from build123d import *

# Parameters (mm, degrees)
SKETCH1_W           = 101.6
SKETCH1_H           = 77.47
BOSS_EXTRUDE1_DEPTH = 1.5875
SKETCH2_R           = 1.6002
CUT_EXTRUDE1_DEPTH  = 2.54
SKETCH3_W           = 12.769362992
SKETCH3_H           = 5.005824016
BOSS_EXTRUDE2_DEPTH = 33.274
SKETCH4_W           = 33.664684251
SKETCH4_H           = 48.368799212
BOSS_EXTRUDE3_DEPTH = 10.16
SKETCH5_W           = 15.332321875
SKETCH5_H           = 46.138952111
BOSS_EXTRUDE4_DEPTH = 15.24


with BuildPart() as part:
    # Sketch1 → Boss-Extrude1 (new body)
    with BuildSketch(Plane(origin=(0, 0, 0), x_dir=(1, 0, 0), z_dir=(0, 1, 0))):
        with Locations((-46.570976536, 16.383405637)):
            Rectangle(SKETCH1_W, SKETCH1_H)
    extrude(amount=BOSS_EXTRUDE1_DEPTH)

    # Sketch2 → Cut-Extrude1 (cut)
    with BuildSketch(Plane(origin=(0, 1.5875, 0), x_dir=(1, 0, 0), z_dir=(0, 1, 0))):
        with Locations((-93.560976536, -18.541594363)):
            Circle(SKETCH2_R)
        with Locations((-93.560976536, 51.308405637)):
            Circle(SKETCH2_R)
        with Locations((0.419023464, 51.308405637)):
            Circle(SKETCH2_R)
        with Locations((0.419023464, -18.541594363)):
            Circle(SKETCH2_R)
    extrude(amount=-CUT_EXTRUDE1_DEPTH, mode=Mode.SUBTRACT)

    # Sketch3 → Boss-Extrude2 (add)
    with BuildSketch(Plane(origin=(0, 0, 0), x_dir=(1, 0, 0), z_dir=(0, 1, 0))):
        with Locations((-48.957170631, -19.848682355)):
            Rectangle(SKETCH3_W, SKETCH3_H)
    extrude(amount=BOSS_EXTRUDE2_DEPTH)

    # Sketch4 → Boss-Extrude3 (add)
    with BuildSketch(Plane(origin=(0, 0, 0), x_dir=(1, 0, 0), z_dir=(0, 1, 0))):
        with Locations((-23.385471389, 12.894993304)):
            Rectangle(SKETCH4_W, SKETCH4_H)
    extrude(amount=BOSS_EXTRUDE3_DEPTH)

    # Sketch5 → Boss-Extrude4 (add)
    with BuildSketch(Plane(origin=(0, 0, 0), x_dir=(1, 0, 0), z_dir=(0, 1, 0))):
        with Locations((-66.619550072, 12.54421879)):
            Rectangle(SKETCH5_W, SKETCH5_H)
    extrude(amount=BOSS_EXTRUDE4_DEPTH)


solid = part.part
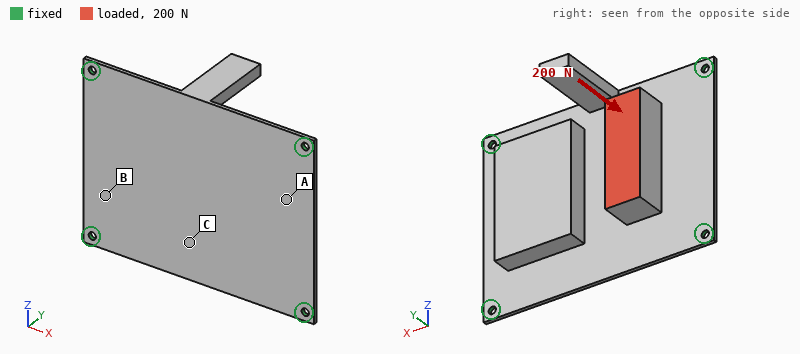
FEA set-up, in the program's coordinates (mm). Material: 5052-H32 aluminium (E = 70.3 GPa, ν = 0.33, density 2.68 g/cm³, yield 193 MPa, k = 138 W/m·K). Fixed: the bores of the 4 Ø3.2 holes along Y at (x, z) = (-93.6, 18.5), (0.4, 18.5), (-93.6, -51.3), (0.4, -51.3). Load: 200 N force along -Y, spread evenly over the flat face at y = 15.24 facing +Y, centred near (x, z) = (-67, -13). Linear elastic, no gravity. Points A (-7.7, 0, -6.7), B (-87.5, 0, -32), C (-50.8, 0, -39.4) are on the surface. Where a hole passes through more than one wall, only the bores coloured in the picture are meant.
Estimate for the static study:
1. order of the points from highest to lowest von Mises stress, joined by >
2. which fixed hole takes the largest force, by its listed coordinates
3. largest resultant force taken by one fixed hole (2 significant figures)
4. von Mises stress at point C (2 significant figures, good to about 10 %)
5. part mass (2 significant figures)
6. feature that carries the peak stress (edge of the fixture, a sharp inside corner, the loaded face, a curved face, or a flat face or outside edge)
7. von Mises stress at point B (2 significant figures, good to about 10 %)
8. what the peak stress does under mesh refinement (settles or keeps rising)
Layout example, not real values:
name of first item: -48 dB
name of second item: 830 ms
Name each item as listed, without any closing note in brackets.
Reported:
order of the points from highest to lowest von Mises stress, joined by >: C > B > A
which fixed hole takes the largest force, by its listed coordinates: (-93.6, 18.5)
largest resultant force taken by one fixed hole: 92 N
von Mises stress at point C: 38 MPa
part mass: 100 g
feature that carries the peak stress: edge of the fixture
von Mises stress at point B: 20 MPa
what the peak stress does under mesh refinement: keeps rising
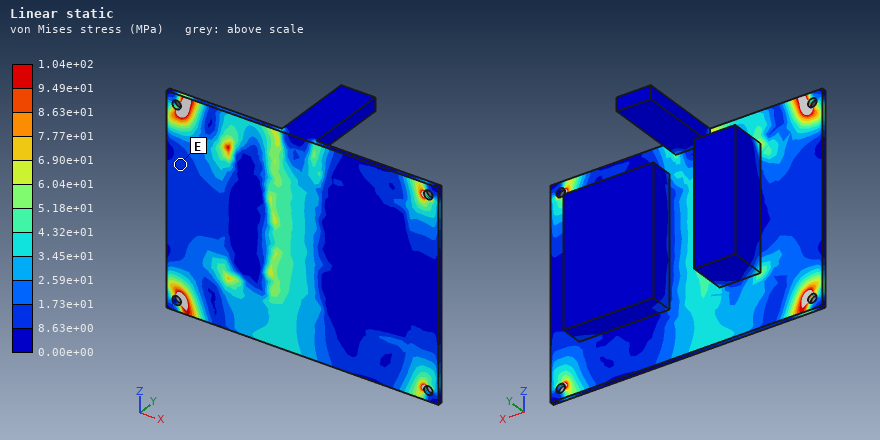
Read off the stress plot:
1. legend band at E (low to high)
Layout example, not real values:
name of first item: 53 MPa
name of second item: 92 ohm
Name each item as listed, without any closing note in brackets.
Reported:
legend band at E: 8.63e+00 to 1.73e+01 MPa
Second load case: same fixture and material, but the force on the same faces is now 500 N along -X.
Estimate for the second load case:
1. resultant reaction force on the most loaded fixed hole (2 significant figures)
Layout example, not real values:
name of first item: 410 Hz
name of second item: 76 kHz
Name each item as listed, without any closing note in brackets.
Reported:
resultant reaction force on the most loaded fixed hole: 170 N
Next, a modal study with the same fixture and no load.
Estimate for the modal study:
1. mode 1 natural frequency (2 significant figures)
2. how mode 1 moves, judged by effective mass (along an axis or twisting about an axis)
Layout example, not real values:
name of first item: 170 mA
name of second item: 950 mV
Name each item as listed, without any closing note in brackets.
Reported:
mode 1 natural frequency: 470 Hz
how mode 1 moves, judged by effective mass: along Y
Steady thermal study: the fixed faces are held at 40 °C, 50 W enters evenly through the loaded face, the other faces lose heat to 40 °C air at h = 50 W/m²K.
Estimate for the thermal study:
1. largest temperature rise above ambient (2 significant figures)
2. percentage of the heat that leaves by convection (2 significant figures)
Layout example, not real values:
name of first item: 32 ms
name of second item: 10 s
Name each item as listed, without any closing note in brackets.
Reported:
largest temperature rise above ambient: 57 K
percentage of the heat that leaves by convection: 54 %
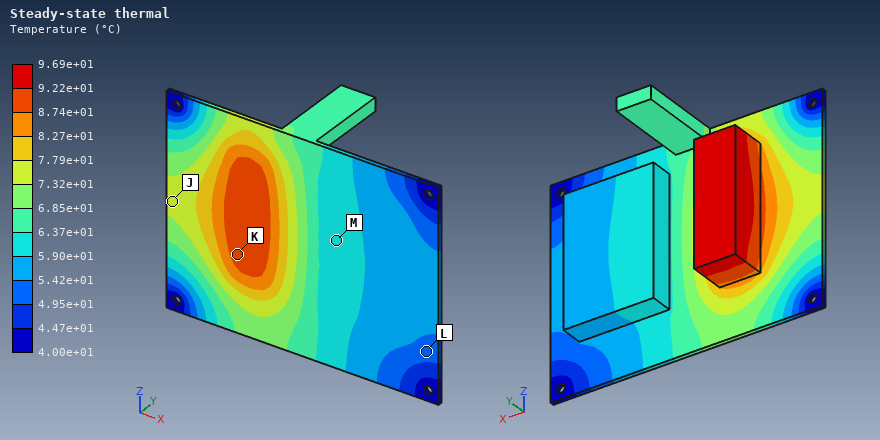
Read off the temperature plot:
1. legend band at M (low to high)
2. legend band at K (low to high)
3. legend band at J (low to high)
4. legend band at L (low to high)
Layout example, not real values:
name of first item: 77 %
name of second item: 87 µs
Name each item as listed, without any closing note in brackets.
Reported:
legend band at M: 5.90e+01 to 6.37e+01 °C
legend band at K: 8.74e+01 to 9.22e+01 °C
legend band at J: 7.32e+01 to 7.79e+01 °C
legend band at L: 4.95e+01 to 5.42e+01 °C
